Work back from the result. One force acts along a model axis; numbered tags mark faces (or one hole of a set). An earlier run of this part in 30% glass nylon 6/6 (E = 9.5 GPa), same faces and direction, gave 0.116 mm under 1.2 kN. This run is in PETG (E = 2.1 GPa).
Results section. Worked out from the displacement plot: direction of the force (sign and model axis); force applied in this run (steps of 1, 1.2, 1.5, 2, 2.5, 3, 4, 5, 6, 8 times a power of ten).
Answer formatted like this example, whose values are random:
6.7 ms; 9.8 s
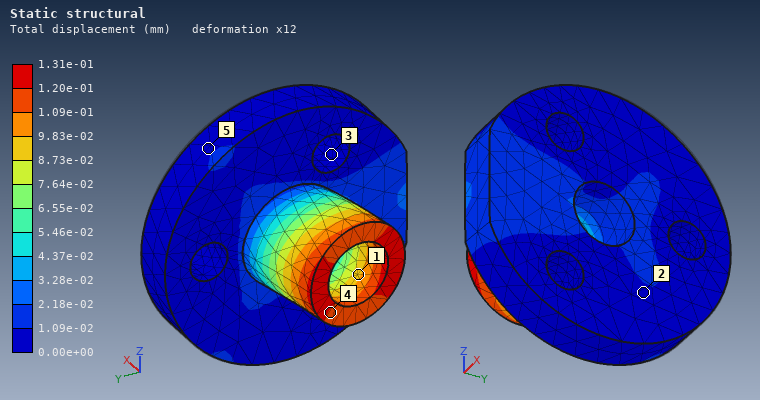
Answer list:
-Y; 300 N
